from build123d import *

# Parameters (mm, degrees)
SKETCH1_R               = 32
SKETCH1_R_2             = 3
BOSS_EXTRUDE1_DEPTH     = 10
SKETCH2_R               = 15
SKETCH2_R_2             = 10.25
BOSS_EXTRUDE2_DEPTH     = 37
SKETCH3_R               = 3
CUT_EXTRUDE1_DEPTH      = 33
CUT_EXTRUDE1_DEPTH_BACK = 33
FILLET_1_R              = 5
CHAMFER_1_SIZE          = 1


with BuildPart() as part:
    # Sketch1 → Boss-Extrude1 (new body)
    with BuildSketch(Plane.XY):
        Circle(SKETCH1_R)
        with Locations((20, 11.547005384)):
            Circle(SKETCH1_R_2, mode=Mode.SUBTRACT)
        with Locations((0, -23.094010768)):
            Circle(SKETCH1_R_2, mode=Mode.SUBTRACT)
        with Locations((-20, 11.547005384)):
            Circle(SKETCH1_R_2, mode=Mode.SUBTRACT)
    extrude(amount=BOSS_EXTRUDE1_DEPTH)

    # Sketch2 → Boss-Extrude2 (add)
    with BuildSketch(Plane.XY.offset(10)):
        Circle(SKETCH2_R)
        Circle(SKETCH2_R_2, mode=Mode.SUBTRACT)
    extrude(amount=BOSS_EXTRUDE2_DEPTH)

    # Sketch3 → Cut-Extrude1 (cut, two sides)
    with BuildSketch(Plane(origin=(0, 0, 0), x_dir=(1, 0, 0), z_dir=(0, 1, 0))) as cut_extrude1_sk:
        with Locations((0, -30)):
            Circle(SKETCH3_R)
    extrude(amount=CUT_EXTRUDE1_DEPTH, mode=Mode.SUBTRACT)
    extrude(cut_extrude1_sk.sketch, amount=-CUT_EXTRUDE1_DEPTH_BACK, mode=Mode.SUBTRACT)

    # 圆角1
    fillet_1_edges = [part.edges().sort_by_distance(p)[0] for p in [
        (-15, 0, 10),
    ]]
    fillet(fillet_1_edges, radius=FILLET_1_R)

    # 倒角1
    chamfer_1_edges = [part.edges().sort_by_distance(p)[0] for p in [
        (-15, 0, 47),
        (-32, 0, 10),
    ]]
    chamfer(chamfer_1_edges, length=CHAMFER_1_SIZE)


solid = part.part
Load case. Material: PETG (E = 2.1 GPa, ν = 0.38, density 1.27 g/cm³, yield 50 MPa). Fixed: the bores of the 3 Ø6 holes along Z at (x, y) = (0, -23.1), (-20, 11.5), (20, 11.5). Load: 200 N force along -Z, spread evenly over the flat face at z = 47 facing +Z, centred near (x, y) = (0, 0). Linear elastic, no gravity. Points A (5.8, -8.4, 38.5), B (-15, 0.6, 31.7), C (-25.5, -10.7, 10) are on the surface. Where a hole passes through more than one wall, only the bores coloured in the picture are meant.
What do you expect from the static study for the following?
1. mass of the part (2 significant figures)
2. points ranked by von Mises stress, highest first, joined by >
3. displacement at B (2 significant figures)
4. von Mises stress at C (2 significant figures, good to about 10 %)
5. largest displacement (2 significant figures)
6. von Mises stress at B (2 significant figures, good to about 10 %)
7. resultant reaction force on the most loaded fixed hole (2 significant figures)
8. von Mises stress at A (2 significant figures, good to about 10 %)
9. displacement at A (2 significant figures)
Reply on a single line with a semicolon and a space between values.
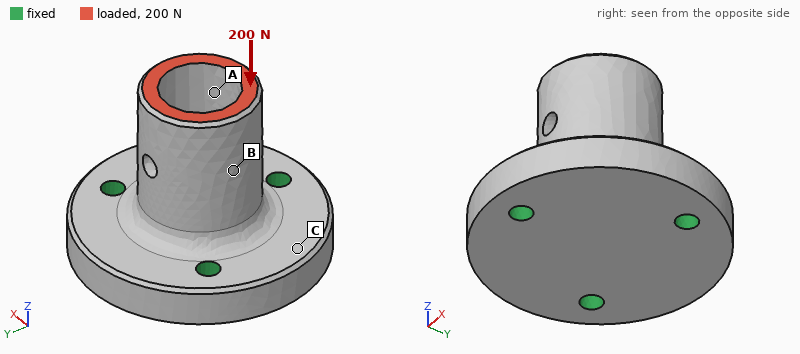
58 g; A > B > C; 11 µm; 0.20 MPa; 16 µm; 0.47 MPa; 69 N; 0.68 MPa; 13 µm
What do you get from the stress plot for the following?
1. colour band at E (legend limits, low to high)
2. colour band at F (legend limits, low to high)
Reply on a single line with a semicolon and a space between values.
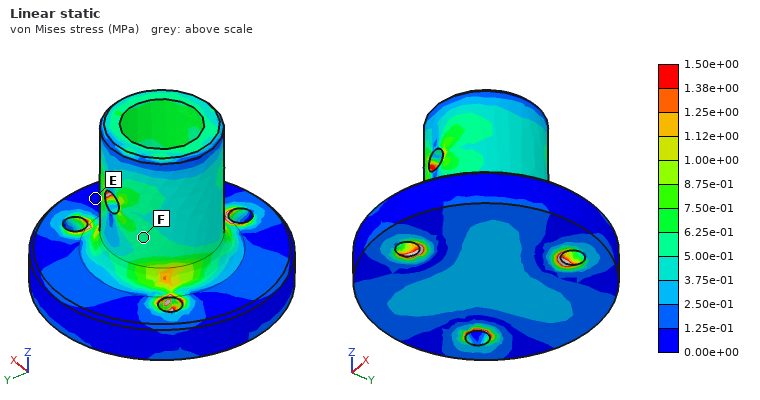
0.00e+00 to 1.25e-01 MPa; 5.00e-01 to 6.25e-01 MPa
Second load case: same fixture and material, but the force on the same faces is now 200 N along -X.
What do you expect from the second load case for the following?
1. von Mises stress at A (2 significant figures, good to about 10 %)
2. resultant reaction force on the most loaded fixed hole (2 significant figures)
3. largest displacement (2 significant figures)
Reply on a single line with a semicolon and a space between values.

2.1 MPa; 210 N; 0.16 mm
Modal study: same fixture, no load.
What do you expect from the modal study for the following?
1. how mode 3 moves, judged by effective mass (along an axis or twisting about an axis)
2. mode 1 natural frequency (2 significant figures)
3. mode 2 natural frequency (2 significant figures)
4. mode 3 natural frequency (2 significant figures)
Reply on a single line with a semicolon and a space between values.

along Z; 2300 Hz; 2400 Hz; 4200 Hz
